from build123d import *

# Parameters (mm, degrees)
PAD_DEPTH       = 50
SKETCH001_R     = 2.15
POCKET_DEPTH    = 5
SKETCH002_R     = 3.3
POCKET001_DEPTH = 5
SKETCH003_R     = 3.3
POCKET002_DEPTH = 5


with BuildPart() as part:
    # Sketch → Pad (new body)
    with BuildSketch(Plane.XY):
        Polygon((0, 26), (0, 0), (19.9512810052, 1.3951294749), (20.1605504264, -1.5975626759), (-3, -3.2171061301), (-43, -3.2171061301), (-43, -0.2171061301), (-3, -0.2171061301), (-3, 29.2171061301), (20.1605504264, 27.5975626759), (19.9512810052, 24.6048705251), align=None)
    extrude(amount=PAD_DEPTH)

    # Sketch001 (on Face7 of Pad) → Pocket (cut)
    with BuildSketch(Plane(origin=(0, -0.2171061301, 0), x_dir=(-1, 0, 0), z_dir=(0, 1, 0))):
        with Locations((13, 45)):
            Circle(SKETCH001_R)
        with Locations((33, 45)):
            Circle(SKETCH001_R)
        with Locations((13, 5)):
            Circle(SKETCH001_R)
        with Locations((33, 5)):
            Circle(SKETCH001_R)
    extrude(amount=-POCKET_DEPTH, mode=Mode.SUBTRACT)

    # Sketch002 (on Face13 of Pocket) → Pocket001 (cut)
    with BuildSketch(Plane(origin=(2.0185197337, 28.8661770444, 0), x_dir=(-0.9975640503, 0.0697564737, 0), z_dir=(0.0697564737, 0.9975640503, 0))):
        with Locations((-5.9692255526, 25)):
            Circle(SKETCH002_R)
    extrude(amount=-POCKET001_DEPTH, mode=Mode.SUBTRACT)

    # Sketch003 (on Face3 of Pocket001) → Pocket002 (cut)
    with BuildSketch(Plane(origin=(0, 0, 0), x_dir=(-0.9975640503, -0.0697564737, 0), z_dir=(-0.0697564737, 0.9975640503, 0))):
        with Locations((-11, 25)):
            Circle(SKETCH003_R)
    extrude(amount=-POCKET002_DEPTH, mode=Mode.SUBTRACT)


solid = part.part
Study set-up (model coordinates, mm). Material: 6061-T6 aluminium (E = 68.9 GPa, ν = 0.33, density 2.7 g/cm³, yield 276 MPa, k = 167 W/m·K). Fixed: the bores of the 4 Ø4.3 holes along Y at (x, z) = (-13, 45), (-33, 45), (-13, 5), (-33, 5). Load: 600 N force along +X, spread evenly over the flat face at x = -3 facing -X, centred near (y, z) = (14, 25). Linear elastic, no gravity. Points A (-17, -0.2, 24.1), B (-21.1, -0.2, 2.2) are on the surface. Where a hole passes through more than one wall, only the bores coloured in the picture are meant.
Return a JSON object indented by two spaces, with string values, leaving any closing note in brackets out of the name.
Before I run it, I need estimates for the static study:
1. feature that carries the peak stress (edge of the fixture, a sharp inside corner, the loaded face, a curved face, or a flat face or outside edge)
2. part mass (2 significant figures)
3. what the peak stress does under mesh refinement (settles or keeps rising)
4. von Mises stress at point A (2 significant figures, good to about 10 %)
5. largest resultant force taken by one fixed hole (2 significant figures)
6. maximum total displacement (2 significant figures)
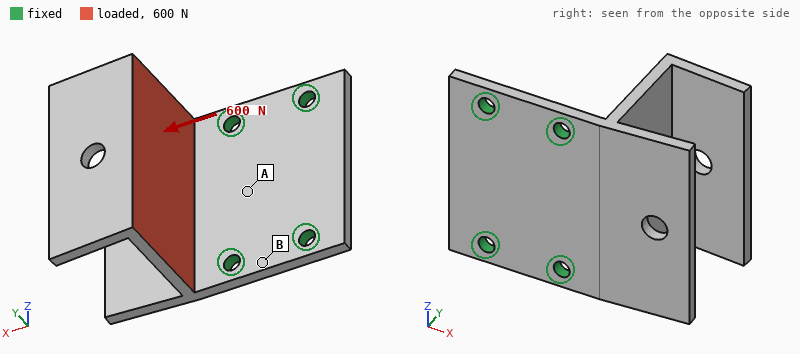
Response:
{
  "feature that carries the peak stress": "edge of the fixture",
  "part mass": "45 g",
  "what the peak stress does under mesh refinement": "keeps rising",
  "von Mises stress at point A": "44 MPa",
  "largest resultant force taken by one fixed hole": "240 N",
  "maximum total displacement": "0.87 mm"
}
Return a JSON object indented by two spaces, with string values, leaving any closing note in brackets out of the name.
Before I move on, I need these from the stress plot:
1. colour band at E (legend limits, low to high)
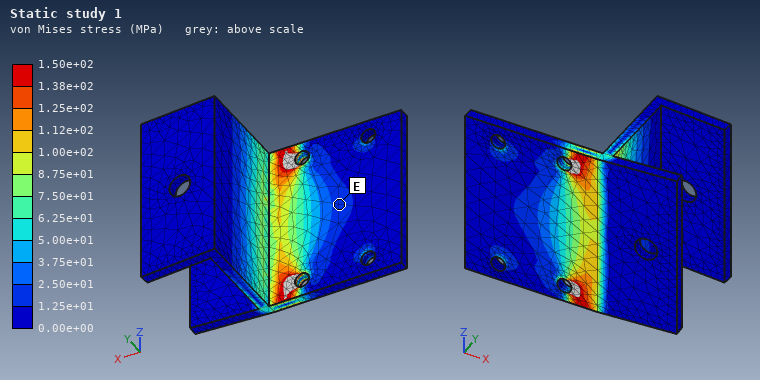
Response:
{
  "colour band at E": "1.25e+01 to 2.50e+01 MPa"
}
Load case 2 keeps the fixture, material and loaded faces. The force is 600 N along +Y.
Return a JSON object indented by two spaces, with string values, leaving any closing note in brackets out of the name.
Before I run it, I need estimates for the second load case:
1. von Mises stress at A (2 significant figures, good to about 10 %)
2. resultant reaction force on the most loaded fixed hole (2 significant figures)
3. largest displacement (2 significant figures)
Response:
{
  "von Mises stress at A": "16 MPa",
  "resultant reaction force on the most loaded fixed hole": "330 N",
  "largest displacement": "0.12 mm"
}
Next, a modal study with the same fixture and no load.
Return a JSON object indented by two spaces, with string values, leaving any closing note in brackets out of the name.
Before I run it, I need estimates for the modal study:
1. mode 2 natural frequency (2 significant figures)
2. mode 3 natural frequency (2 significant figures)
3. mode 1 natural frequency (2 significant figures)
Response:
{
  "mode 2 natural frequency": "2200 Hz",
  "mode 3 natural frequency": "3000 Hz",
  "mode 1 natural frequency": "860 Hz"
}
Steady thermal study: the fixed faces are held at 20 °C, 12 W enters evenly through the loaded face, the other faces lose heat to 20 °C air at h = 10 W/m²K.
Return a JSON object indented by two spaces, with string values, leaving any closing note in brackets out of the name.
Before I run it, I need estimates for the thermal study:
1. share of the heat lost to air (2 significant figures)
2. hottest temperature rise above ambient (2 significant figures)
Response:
{
  "share of the heat lost to air": "5.9 %",
  "hottest temperature rise above ambient": "13 K"
}
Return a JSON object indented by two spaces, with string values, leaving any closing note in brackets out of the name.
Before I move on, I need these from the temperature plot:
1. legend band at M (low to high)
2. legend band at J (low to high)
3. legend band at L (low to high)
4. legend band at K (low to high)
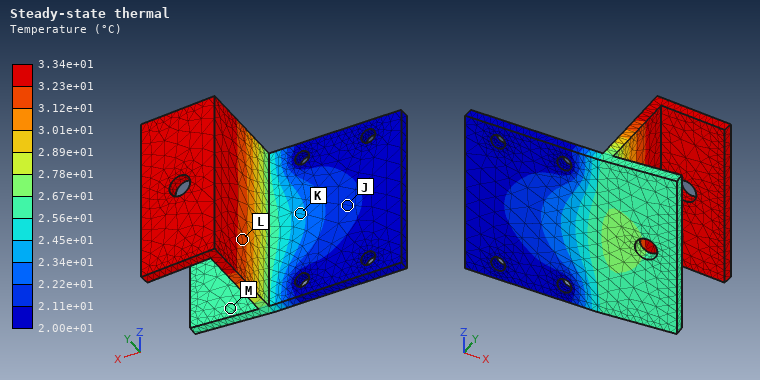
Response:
{
  "legend band at M": "2.56e+01 to 2.67e+01 °C",
  "legend band at J": "2.11e+01 to 2.22e+01 °C",
  "legend band at L": "3.12e+01 to 3.23e+01 °C",
  "legend band at K": "2.34e+01 to 2.45e+01 °C"
}
